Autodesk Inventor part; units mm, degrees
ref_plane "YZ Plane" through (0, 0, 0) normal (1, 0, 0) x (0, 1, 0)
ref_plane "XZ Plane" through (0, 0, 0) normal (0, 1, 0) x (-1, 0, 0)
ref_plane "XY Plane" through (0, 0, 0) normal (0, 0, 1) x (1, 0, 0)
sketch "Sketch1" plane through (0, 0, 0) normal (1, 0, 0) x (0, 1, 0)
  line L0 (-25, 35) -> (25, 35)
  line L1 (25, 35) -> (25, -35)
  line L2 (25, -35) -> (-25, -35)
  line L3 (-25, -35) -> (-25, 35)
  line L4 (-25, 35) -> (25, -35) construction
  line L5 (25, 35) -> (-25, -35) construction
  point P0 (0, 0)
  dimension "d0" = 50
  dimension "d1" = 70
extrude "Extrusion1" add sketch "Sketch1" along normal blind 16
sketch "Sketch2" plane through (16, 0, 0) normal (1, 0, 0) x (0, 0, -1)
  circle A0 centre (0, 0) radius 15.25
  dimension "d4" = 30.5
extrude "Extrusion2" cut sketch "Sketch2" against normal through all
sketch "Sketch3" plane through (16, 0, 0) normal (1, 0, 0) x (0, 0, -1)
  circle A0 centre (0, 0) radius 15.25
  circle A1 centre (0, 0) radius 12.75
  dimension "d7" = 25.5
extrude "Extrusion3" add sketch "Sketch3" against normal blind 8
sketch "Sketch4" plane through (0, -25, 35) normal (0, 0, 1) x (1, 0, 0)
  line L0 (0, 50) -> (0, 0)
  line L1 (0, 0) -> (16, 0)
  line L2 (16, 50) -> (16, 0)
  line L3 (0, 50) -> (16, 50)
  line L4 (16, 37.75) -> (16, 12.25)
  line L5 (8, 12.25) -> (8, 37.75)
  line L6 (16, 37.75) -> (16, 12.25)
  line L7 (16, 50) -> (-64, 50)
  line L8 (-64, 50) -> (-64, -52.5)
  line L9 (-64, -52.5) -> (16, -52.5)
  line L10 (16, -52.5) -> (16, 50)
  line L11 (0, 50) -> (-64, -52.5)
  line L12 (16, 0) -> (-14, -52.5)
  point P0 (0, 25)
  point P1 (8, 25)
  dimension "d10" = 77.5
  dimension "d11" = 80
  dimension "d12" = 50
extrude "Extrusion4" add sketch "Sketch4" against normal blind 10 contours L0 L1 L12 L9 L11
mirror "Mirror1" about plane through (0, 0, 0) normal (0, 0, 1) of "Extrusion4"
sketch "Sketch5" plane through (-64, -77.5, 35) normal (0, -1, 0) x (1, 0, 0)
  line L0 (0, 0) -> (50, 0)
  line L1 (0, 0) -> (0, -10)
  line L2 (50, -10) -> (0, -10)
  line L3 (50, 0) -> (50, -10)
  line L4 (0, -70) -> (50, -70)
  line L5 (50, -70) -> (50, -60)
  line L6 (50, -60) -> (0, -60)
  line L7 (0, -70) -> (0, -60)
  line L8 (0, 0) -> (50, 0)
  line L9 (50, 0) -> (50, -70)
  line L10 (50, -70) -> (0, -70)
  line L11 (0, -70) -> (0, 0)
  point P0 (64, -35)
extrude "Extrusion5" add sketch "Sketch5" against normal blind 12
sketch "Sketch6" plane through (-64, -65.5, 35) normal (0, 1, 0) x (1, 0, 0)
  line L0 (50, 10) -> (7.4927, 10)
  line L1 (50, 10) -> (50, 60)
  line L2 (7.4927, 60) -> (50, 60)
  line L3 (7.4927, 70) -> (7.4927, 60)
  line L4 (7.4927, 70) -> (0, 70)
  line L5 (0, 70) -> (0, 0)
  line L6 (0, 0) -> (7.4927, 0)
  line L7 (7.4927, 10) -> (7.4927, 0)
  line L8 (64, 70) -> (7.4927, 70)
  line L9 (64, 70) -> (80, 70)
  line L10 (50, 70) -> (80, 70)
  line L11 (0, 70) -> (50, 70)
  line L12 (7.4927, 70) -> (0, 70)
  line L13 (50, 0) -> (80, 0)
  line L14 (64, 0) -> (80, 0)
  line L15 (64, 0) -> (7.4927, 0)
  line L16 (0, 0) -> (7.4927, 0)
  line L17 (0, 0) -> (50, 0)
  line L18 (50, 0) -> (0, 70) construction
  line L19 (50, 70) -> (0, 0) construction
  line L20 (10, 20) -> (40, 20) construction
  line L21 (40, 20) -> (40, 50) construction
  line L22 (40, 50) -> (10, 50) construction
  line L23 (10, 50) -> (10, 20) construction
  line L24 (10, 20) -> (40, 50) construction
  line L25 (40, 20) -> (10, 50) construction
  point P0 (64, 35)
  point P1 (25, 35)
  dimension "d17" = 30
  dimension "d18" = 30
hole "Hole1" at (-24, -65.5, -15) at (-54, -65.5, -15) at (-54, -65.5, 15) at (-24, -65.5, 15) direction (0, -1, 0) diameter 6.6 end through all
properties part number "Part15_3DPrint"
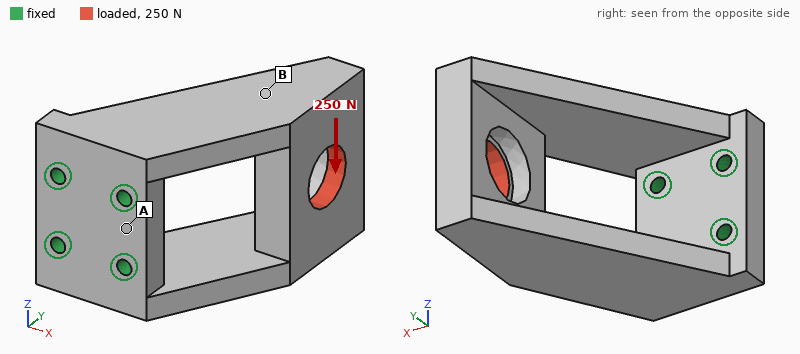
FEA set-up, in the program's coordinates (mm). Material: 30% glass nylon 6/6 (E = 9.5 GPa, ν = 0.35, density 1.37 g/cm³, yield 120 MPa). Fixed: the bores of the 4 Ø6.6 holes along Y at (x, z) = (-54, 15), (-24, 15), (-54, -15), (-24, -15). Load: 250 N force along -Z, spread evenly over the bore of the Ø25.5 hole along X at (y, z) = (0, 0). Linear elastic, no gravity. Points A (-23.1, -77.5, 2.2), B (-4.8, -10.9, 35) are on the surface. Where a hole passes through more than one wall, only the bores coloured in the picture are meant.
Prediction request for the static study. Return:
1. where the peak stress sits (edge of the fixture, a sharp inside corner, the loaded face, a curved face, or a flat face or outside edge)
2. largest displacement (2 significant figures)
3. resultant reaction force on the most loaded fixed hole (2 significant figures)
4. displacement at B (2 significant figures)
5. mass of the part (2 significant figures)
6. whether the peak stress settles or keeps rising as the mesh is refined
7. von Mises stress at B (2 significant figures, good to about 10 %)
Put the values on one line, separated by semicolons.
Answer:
edge of the fixture; 0.19 mm; 260 N; 0.15 mm; 190 g; keeps rising; 2.5 MPa
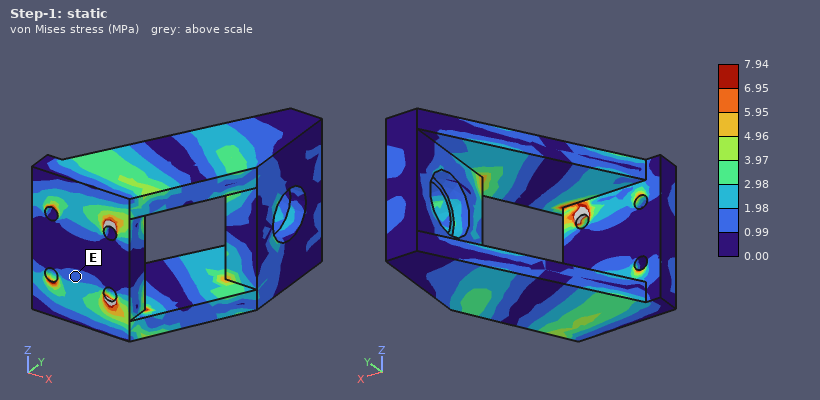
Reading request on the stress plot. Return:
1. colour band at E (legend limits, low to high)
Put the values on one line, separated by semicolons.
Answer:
0.99 to 1.98 MPa
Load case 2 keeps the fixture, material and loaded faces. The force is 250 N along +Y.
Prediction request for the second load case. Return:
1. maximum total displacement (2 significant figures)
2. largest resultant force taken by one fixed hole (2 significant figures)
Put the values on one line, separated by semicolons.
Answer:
81 µm; 240 N
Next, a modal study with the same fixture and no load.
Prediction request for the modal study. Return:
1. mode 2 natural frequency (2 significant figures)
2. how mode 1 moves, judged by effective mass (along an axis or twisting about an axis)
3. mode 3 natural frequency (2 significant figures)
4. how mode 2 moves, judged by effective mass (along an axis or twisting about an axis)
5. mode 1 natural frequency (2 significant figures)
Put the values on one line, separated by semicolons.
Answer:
850 Hz; along Z; 1500 Hz; along X; 640 Hz
